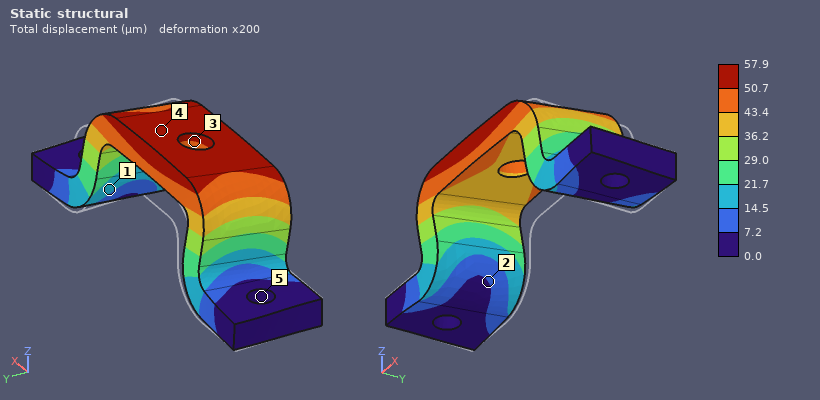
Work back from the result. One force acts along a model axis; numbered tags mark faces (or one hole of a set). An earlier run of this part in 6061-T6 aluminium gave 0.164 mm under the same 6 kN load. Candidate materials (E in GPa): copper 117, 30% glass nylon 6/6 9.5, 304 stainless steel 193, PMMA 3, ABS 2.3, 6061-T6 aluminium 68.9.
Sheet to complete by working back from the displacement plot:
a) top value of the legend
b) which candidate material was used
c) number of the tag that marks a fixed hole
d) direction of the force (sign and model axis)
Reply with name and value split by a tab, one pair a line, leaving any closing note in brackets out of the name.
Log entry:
top value of the legend	57.9 µm
which candidate material was used	304 stainless steel
number of the tag that marks a fixed hole	5
direction of the force	-Y
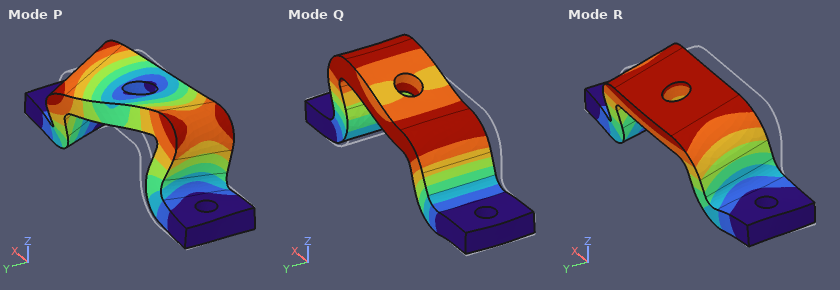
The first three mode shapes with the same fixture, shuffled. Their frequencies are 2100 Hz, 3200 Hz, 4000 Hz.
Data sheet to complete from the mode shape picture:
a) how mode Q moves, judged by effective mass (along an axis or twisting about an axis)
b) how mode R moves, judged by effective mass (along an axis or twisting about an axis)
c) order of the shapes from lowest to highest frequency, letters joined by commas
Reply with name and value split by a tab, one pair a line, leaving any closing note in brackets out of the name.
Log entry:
how mode Q moves, judged by effective mass	along X
how mode R moves, judged by effective mass	along Y
order of the shapes from lowest to highest frequency, letters joined by commas	R, Q, P
